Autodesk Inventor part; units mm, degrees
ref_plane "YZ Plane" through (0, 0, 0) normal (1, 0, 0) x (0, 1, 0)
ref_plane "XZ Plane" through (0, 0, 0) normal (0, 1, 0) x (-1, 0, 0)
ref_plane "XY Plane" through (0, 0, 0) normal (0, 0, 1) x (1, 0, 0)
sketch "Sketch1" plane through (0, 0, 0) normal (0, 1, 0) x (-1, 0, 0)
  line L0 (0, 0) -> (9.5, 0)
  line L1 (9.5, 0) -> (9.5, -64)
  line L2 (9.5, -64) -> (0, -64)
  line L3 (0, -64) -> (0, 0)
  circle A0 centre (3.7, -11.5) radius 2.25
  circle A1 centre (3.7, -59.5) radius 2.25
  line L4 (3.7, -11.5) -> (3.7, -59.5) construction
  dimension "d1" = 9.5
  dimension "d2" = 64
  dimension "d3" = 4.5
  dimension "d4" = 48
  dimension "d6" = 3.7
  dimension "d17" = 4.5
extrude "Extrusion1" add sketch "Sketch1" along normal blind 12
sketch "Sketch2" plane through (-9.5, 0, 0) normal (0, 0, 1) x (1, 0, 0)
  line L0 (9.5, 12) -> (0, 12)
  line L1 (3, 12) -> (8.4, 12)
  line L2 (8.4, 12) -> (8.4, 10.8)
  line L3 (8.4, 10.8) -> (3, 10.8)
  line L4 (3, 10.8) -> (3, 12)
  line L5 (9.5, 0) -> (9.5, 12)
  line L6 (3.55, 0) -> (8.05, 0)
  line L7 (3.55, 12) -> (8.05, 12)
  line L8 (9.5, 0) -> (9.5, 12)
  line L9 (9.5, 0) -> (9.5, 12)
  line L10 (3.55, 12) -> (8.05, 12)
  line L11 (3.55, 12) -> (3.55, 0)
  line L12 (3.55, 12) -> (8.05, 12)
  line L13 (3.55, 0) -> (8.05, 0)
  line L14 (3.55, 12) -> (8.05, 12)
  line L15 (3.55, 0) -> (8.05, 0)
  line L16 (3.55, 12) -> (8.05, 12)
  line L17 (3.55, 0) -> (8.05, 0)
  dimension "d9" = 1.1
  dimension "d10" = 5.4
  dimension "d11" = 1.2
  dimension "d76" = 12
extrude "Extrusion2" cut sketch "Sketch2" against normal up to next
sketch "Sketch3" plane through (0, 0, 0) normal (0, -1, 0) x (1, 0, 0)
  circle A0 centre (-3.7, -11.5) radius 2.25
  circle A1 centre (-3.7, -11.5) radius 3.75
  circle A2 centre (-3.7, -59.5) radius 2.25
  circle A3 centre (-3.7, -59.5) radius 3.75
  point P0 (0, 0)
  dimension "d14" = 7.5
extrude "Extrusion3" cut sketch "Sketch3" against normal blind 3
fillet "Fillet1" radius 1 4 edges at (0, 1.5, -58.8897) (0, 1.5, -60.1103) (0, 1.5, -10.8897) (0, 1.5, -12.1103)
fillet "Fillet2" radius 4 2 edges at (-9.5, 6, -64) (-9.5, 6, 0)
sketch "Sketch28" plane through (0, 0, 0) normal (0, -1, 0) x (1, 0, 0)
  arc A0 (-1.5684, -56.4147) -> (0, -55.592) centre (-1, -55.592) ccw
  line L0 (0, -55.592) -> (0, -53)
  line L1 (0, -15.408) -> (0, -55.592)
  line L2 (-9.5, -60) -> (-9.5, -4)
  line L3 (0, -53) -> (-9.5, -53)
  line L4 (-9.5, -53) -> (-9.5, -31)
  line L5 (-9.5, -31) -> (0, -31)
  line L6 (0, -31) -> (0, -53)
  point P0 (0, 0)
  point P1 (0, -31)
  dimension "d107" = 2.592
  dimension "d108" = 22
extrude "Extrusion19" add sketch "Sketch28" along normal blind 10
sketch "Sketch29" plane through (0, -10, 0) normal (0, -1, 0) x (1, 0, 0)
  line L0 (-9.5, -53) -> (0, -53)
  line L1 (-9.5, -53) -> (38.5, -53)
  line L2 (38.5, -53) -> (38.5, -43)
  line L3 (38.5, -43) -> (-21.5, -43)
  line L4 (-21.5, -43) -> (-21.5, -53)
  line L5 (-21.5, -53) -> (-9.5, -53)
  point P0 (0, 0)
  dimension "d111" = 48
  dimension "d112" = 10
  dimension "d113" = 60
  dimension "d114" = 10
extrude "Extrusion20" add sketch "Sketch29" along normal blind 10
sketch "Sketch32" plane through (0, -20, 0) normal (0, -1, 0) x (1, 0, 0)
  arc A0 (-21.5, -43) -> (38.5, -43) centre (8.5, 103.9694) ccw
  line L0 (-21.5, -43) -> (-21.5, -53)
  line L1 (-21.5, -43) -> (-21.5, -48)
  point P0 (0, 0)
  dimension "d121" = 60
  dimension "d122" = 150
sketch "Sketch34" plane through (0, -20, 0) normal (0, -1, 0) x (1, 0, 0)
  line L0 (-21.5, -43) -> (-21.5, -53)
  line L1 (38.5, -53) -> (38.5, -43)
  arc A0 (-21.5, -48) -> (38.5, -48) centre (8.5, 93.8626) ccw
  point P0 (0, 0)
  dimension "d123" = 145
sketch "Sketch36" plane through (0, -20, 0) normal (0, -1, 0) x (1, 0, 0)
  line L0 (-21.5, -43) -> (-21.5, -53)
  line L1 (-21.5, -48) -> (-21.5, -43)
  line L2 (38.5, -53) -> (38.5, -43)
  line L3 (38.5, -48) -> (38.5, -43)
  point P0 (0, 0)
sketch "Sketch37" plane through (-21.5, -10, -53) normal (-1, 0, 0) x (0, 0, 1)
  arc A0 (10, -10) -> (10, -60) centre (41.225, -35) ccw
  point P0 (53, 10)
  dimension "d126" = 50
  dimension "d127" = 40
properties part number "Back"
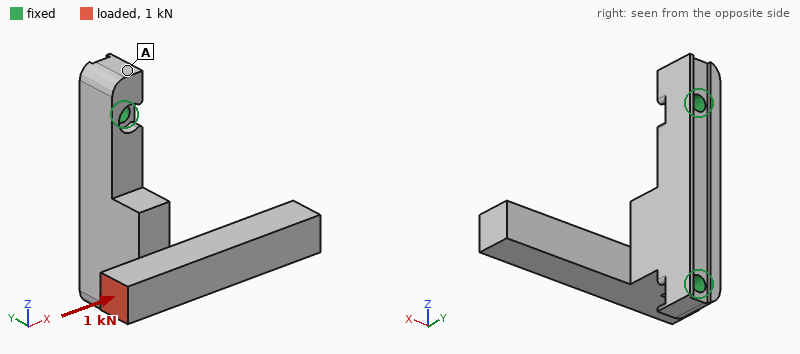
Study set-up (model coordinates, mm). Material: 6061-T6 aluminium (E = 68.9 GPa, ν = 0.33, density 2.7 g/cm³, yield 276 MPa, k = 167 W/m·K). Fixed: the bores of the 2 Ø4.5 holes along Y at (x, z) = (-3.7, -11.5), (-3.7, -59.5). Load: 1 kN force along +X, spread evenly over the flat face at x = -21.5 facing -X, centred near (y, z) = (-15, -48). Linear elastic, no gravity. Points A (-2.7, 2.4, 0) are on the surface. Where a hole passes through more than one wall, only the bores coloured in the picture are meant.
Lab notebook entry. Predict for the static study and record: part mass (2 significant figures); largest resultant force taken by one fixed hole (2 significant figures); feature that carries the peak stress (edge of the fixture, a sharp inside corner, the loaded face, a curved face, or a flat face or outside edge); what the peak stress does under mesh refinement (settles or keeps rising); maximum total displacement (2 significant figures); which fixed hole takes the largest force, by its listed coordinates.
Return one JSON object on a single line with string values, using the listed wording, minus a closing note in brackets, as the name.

{"part mass": "39 g", "largest resultant force taken by one fixed hole": "840 N", "feature that carries the peak stress": "edge of the fixture", "what the peak stress does under mesh refinement": "keeps rising", "maximum total displacement": "0.32 mm", "which fixed hole takes the largest force, by its listed coordinates": "(-3.7, -59.5)"}
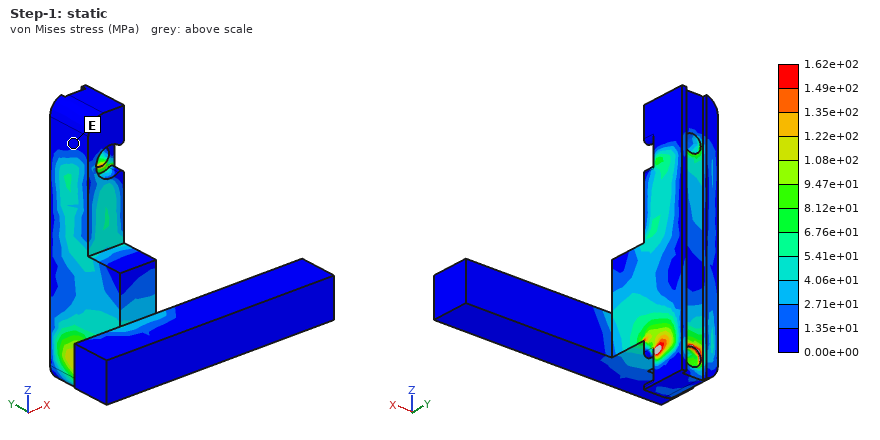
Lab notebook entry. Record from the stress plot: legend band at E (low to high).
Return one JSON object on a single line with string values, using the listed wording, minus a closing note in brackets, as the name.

{"legend band at E": "0.00e+00 to 1.35e+01 MPa"}
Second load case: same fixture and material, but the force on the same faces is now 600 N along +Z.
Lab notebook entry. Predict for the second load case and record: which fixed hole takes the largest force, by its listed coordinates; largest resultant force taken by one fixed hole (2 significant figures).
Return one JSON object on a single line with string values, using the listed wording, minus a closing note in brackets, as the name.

{"which fixed hole takes the largest force, by its listed coordinates": "(-3.7, -11.5)", "largest resultant force taken by one fixed hole": "540 N"}
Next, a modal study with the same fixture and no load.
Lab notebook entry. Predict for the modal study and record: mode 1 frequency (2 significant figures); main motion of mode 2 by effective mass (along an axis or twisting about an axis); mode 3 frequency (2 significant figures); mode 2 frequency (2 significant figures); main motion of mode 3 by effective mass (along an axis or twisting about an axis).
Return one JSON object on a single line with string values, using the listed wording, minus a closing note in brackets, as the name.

{"mode 1 frequency": "2100 Hz", "main motion of mode 2 by effective mass": "along Z", "mode 3 frequency": "5600 Hz", "mode 2 frequency": "2900 Hz", "main motion of mode 3 by effective mass": "along X"}
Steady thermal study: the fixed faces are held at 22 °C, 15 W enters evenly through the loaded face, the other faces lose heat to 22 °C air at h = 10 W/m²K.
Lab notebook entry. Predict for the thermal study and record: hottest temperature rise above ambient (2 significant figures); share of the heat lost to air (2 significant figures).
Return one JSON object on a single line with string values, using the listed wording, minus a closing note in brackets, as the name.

{"hottest temperature rise above ambient": "29 K", "share of the heat lost to air": "3.6 %"}
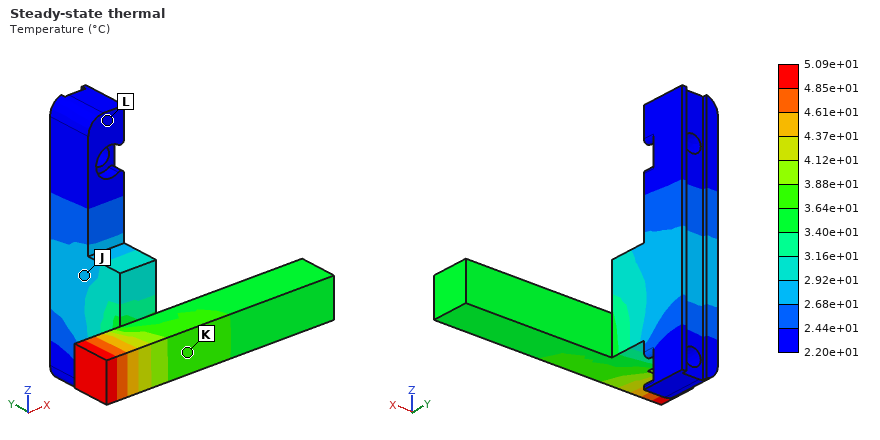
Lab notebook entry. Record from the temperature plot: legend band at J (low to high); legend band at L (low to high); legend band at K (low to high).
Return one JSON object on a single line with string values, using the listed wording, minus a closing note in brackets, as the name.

{"legend band at J": "2.68e+01 to 2.92e+01 °C", "legend band at L": "2.20e+01 to 2.44e+01 °C", "legend band at K": "3.64e+01 to 3.88e+01 °C"}
